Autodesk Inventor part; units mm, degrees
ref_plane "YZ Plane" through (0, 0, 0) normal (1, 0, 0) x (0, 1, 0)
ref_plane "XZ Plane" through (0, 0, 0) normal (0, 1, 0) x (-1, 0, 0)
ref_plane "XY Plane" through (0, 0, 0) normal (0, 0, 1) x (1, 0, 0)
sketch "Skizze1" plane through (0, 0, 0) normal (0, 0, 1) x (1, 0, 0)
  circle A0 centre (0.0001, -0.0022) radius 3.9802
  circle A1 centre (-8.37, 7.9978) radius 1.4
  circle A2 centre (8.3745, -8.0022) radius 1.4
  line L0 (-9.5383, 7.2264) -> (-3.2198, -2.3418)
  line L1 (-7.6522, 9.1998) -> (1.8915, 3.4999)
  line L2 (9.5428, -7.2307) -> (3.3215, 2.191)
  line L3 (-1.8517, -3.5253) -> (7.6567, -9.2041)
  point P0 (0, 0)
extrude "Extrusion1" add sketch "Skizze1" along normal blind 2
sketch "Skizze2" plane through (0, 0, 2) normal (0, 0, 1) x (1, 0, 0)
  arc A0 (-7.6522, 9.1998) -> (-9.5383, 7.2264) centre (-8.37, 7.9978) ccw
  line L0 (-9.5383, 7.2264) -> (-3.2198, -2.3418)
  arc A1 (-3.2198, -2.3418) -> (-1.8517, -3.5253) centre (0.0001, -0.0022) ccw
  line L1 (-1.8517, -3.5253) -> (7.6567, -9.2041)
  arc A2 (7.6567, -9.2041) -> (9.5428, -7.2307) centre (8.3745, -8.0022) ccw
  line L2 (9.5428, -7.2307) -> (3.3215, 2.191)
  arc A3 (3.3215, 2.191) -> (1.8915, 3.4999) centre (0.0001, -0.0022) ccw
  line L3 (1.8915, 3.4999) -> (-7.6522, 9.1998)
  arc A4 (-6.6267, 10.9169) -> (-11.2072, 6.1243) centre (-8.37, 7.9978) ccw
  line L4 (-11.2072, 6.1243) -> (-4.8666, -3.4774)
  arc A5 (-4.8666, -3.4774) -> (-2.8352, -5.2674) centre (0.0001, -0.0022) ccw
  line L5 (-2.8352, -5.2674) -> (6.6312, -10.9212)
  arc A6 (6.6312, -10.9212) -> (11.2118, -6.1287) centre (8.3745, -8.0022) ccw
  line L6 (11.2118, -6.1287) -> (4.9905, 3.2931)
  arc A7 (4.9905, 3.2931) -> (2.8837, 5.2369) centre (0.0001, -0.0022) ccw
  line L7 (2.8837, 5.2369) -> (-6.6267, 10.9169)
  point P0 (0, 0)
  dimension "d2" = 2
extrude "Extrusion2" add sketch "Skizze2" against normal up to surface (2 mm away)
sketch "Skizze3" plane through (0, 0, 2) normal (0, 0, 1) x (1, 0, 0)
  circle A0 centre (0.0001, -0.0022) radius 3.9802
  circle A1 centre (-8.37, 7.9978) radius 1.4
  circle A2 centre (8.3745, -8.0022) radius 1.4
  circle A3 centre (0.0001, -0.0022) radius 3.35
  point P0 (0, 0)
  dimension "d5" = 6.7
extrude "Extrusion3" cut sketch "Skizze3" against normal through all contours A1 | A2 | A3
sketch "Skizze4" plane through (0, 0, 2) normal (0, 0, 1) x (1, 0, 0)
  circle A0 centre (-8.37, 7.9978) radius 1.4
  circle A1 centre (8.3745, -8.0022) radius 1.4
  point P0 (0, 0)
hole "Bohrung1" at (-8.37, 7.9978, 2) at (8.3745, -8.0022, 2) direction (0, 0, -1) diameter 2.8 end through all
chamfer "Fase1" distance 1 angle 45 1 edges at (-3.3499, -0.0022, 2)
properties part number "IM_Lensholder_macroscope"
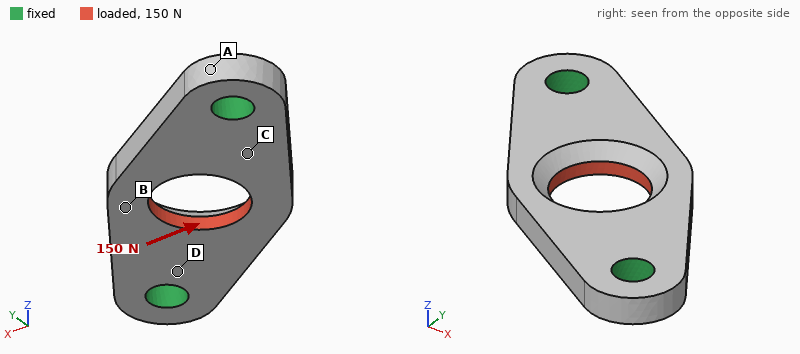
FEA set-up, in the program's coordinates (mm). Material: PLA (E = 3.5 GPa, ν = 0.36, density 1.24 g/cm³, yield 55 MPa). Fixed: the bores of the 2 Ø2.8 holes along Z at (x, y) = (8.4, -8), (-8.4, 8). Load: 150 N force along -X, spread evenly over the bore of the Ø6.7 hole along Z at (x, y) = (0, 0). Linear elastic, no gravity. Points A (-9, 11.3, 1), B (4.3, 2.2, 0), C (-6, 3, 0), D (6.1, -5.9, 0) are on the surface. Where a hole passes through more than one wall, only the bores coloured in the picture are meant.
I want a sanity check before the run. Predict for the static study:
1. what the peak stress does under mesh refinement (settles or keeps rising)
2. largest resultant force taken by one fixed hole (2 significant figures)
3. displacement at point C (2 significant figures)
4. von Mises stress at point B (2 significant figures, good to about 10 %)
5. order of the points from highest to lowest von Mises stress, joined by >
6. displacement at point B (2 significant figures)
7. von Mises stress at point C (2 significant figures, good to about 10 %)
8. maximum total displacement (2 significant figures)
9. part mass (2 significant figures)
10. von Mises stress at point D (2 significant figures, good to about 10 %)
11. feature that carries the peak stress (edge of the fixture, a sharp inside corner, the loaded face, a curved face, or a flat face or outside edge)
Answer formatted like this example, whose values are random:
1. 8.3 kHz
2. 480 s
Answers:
1. keeps rising
2. 75 N
3. 31 µm
4. 6.8 MPa
5. D > C > B > A
6. 61 µm
7. 9.6 MPa
8. 67 µm
9. 0.51 g
10. 13 MPa
11. edge of the fixture
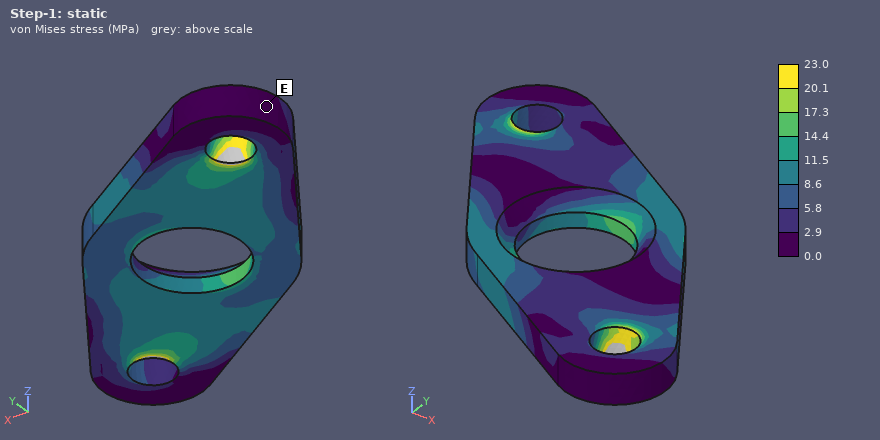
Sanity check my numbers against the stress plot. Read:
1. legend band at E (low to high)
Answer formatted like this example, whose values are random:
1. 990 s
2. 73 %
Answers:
1. 0.0 to 2.9 MPa
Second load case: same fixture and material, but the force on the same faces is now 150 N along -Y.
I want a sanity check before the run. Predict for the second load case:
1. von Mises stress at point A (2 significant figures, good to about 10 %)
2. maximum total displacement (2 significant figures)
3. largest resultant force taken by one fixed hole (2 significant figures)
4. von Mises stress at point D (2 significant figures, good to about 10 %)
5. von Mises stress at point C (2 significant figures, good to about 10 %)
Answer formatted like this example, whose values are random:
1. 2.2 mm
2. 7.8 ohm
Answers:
1. 2.2 MPa
2. 70 µm
3. 75 N
4. 13 MPa
5. 11 MPa
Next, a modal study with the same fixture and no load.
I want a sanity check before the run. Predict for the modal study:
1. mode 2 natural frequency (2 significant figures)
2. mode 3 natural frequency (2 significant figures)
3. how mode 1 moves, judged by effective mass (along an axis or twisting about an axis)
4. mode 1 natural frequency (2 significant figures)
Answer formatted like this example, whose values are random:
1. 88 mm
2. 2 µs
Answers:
1. 7800 Hz
2. 15 kHz
3. along Z
4. 6700 Hz
